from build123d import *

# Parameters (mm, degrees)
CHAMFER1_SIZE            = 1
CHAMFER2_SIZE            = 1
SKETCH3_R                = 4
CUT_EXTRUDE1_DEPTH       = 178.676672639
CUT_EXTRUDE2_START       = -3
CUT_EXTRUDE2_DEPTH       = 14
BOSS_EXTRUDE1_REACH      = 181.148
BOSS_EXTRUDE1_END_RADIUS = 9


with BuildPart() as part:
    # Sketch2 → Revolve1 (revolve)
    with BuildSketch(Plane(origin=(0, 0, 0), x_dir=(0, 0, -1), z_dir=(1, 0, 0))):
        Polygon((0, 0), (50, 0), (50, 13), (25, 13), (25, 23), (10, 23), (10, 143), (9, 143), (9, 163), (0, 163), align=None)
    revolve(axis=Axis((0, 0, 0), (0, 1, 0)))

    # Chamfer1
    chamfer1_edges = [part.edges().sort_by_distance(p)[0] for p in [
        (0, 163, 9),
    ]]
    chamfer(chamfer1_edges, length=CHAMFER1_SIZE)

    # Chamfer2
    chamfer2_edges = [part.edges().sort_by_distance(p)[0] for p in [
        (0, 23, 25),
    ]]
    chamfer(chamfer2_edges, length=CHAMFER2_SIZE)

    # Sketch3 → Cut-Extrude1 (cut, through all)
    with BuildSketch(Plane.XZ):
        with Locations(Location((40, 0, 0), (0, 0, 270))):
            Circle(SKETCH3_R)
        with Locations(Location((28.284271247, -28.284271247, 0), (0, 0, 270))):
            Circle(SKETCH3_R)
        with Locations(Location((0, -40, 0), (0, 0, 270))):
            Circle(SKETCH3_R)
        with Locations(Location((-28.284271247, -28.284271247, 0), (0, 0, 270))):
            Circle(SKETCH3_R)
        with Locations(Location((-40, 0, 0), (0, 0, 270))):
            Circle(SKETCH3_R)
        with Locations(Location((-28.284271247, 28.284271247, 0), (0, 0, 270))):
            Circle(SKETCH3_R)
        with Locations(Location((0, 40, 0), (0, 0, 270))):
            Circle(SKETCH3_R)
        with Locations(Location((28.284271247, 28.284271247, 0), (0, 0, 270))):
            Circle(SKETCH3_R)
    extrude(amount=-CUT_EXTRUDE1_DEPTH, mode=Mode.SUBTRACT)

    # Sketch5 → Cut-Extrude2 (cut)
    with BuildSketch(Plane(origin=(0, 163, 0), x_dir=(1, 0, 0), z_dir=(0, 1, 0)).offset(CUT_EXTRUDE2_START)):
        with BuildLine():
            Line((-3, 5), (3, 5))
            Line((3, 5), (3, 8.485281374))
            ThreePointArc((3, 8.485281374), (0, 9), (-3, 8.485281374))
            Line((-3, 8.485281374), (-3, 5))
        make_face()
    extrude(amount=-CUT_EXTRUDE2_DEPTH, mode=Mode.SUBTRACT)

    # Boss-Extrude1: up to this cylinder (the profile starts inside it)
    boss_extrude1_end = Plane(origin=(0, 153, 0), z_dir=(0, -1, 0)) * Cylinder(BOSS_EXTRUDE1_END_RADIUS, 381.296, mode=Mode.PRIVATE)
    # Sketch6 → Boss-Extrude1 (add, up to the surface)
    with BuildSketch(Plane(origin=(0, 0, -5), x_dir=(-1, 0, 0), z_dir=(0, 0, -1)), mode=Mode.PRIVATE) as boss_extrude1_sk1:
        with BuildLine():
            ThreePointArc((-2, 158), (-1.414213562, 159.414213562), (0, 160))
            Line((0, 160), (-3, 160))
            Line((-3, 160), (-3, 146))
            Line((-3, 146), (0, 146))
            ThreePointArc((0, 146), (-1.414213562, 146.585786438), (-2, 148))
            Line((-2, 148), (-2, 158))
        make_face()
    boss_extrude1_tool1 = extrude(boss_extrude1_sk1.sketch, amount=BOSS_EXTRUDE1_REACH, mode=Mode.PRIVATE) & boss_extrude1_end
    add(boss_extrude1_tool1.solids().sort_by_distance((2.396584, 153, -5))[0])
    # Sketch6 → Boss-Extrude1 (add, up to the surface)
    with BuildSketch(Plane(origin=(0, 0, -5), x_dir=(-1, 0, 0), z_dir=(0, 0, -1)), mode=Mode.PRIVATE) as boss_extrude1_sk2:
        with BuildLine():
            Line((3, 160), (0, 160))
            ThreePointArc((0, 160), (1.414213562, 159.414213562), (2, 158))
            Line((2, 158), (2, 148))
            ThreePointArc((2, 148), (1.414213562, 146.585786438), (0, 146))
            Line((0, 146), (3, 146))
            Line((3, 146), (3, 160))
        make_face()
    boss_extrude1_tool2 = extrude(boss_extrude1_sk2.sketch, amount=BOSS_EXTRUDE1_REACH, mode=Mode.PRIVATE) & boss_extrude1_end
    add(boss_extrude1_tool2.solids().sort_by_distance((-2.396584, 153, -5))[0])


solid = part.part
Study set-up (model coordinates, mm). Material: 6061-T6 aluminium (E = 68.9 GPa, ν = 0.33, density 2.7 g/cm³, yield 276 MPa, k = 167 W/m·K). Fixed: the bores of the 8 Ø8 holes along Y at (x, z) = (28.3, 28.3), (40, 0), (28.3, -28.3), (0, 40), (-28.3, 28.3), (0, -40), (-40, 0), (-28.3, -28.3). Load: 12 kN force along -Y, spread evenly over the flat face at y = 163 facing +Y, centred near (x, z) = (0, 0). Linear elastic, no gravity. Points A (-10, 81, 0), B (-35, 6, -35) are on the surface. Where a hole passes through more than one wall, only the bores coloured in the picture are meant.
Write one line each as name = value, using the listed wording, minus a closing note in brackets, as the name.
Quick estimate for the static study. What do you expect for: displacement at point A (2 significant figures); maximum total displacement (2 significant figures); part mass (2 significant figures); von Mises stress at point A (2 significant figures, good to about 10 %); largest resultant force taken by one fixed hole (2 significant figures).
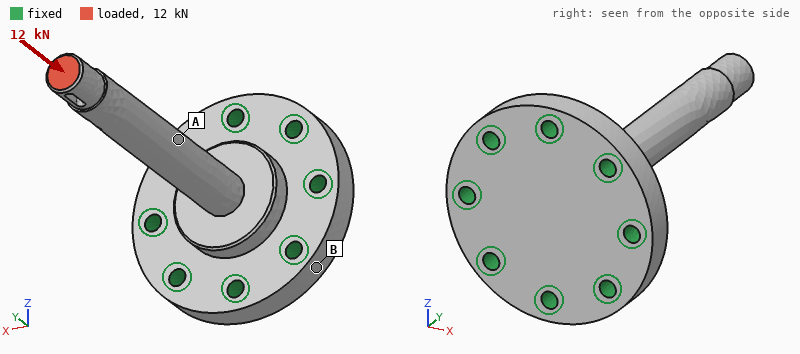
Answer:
displacement at point A = 46 µm
maximum total displacement = 99 µm
part mass = 430 g
von Mises stress at point A = 38 MPa
largest resultant force taken by one fixed hole = 1.8 kN
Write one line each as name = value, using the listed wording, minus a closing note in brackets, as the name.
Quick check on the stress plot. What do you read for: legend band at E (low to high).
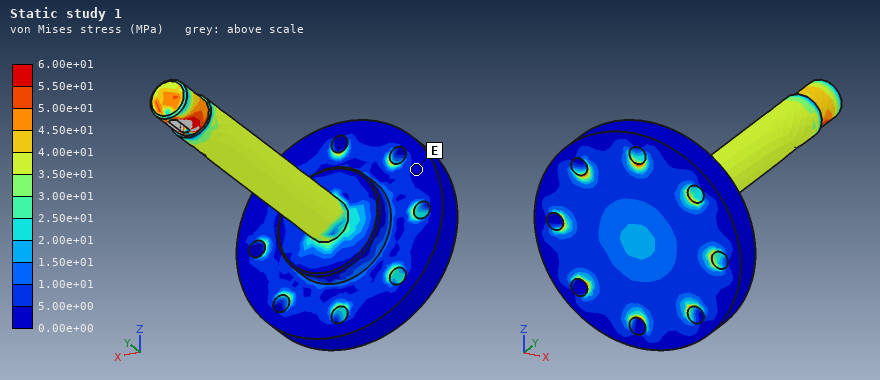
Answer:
legend band at E = 0.00e+00 to 5.00e+00 MPa
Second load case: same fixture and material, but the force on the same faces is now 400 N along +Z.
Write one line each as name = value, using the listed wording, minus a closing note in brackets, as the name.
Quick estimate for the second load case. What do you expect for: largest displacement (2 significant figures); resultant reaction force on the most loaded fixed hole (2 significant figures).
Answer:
largest displacement = 0.76 mm
resultant reaction force on the most loaded fixed hole = 490 N
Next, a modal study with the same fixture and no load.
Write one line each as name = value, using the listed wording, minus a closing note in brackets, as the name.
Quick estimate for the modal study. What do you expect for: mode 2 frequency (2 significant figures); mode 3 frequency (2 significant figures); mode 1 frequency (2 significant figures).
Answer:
mode 2 frequency = 700 Hz
mode 3 frequency = 4100 Hz
mode 1 frequency = 700 Hz
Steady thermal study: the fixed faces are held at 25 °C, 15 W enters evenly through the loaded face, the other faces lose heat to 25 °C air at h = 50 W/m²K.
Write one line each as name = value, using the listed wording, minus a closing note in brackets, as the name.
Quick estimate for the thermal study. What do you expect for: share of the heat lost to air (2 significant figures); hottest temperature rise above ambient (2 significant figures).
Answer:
share of the heat lost to air = 44 %
hottest temperature rise above ambient = 32 K
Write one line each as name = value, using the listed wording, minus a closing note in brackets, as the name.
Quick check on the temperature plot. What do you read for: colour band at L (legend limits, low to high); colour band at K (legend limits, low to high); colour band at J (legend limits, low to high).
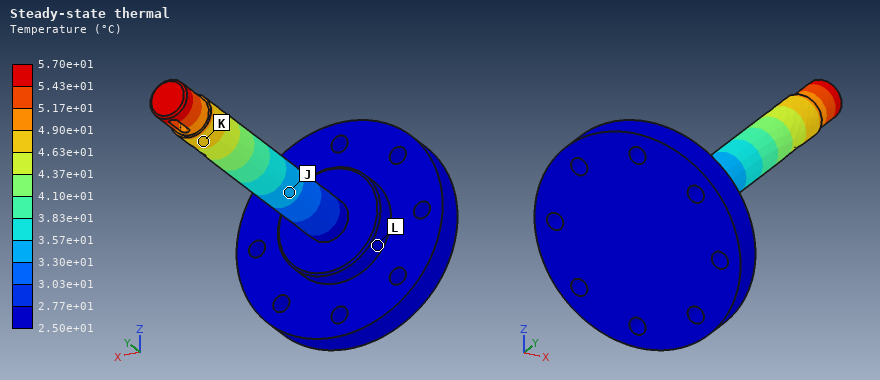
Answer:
colour band at L = 2.50e+01 to 2.77e+01 °C
colour band at K = 4.63e+01 to 4.90e+01 °C
colour band at J = 3.30e+01 to 3.57e+01 °C
